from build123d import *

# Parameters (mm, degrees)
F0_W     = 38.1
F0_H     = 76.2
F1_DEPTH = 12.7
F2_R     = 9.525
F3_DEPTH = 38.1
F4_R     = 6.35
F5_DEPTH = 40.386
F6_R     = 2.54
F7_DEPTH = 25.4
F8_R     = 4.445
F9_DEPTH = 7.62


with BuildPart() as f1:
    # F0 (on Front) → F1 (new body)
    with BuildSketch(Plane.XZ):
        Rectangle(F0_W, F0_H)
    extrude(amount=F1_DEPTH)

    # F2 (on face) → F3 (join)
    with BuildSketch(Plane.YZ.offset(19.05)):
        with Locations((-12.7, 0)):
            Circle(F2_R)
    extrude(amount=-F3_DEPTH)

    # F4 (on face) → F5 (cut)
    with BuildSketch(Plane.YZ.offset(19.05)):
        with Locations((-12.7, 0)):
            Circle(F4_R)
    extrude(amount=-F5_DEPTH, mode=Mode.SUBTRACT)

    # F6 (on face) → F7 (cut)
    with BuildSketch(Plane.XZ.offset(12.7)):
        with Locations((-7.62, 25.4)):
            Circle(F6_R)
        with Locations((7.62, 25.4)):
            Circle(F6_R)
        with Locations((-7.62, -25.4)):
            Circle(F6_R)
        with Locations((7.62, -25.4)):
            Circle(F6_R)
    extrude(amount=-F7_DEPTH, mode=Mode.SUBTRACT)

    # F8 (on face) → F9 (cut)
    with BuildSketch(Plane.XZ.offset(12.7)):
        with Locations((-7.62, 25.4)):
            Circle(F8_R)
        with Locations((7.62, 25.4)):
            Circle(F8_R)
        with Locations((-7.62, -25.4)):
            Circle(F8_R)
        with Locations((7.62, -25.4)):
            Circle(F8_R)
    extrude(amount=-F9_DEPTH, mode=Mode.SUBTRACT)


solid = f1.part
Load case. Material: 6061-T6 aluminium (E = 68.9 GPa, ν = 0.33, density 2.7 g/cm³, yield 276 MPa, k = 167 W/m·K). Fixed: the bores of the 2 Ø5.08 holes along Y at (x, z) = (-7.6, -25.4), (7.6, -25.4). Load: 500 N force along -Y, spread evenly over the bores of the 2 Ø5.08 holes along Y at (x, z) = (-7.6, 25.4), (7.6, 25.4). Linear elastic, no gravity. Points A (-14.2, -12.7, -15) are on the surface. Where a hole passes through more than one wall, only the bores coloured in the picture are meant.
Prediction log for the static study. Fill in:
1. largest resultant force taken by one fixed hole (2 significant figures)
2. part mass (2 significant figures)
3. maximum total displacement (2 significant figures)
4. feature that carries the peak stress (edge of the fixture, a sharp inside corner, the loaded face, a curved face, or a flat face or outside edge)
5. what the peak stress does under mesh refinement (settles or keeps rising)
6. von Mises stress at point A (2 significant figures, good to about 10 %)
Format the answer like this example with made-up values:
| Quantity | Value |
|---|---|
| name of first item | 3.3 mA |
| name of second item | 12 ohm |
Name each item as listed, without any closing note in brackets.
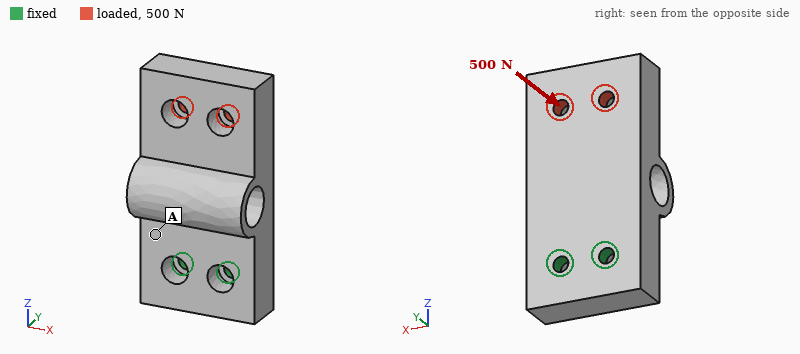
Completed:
| Quantity | Value |
|---|---|
| largest resultant force taken by one fixed hole | 280 N |
| part mass | 95 g |
| maximum total displacement | 0.19 mm |
| feature that carries the peak stress | edge of the fixture |
| what the peak stress does under mesh refinement | keeps rising |
| von Mises stress at point A | 20 MPa |
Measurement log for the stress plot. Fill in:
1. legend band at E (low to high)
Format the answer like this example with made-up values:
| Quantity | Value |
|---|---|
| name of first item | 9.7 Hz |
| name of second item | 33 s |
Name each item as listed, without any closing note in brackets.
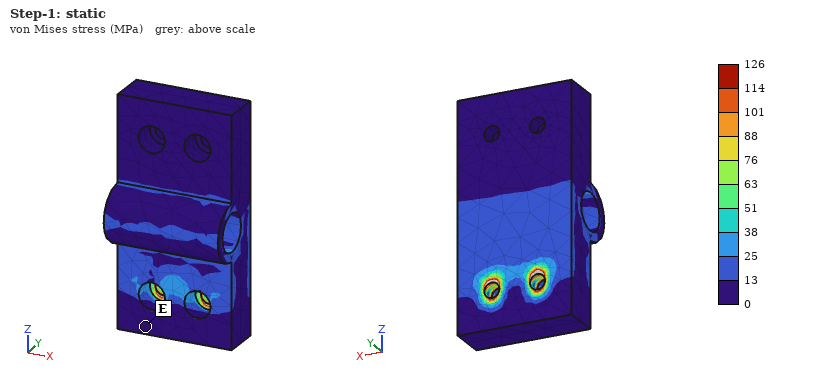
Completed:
| Quantity | Value |
|---|---|
| legend band at E | 0 to 13 MPa |
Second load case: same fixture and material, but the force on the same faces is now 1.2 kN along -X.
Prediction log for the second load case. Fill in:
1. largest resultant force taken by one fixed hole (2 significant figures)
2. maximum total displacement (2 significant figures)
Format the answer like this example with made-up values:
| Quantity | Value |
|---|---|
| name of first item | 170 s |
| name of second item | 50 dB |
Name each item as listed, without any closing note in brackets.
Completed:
| Quantity | Value |
|---|---|
| largest resultant force taken by one fixed hole | 3.3 kN |
| maximum total displacement | 64 µm |
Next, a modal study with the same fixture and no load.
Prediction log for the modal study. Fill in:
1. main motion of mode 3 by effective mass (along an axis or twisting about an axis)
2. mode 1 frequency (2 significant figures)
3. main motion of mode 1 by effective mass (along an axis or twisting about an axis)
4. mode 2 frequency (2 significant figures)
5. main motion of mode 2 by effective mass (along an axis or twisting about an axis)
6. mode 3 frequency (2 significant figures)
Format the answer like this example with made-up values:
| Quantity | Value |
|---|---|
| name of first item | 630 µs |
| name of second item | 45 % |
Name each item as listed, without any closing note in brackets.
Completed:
| Quantity | Value |
|---|---|
| main motion of mode 3 by effective mass | twisting about Z |
| mode 1 frequency | 1500 Hz |
| main motion of mode 1 by effective mass | along Y |
| mode 2 frequency | 4000 Hz |
| main motion of mode 2 by effective mass | along X |
| mode 3 frequency | 6700 Hz |
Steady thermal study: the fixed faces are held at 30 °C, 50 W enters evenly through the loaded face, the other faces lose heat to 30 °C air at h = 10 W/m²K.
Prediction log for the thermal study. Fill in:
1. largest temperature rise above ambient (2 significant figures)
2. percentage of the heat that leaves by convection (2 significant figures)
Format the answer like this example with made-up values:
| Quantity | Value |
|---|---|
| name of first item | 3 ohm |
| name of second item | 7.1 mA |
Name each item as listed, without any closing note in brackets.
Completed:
| Quantity | Value |
|---|---|
| largest temperature rise above ambient | 44 K |
| percentage of the heat that leaves by convection | 4.7 % |
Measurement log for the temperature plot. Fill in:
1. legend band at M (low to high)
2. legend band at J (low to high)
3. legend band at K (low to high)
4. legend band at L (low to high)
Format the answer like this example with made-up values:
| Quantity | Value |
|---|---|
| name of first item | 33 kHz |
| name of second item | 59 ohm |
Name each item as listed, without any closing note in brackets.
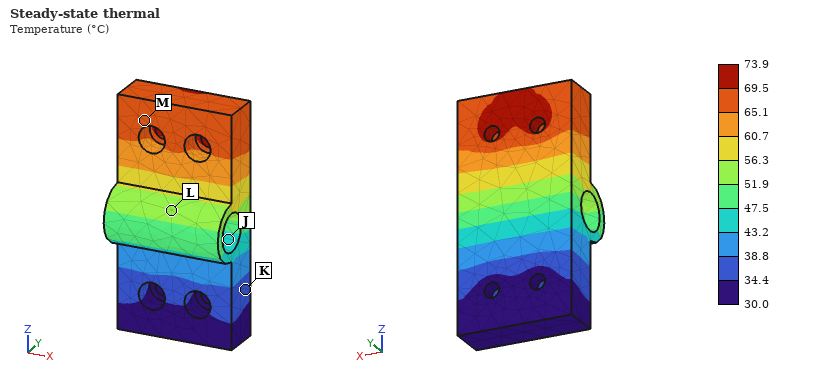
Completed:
| Quantity | Value |
|---|---|
| legend band at M | 65.1 to 69.5 °C |
| legend band at J | 43.2 to 47.5 °C |
| legend band at K | 34.4 to 38.8 °C |
| legend band at L | 51.9 to 56.3 °C |
